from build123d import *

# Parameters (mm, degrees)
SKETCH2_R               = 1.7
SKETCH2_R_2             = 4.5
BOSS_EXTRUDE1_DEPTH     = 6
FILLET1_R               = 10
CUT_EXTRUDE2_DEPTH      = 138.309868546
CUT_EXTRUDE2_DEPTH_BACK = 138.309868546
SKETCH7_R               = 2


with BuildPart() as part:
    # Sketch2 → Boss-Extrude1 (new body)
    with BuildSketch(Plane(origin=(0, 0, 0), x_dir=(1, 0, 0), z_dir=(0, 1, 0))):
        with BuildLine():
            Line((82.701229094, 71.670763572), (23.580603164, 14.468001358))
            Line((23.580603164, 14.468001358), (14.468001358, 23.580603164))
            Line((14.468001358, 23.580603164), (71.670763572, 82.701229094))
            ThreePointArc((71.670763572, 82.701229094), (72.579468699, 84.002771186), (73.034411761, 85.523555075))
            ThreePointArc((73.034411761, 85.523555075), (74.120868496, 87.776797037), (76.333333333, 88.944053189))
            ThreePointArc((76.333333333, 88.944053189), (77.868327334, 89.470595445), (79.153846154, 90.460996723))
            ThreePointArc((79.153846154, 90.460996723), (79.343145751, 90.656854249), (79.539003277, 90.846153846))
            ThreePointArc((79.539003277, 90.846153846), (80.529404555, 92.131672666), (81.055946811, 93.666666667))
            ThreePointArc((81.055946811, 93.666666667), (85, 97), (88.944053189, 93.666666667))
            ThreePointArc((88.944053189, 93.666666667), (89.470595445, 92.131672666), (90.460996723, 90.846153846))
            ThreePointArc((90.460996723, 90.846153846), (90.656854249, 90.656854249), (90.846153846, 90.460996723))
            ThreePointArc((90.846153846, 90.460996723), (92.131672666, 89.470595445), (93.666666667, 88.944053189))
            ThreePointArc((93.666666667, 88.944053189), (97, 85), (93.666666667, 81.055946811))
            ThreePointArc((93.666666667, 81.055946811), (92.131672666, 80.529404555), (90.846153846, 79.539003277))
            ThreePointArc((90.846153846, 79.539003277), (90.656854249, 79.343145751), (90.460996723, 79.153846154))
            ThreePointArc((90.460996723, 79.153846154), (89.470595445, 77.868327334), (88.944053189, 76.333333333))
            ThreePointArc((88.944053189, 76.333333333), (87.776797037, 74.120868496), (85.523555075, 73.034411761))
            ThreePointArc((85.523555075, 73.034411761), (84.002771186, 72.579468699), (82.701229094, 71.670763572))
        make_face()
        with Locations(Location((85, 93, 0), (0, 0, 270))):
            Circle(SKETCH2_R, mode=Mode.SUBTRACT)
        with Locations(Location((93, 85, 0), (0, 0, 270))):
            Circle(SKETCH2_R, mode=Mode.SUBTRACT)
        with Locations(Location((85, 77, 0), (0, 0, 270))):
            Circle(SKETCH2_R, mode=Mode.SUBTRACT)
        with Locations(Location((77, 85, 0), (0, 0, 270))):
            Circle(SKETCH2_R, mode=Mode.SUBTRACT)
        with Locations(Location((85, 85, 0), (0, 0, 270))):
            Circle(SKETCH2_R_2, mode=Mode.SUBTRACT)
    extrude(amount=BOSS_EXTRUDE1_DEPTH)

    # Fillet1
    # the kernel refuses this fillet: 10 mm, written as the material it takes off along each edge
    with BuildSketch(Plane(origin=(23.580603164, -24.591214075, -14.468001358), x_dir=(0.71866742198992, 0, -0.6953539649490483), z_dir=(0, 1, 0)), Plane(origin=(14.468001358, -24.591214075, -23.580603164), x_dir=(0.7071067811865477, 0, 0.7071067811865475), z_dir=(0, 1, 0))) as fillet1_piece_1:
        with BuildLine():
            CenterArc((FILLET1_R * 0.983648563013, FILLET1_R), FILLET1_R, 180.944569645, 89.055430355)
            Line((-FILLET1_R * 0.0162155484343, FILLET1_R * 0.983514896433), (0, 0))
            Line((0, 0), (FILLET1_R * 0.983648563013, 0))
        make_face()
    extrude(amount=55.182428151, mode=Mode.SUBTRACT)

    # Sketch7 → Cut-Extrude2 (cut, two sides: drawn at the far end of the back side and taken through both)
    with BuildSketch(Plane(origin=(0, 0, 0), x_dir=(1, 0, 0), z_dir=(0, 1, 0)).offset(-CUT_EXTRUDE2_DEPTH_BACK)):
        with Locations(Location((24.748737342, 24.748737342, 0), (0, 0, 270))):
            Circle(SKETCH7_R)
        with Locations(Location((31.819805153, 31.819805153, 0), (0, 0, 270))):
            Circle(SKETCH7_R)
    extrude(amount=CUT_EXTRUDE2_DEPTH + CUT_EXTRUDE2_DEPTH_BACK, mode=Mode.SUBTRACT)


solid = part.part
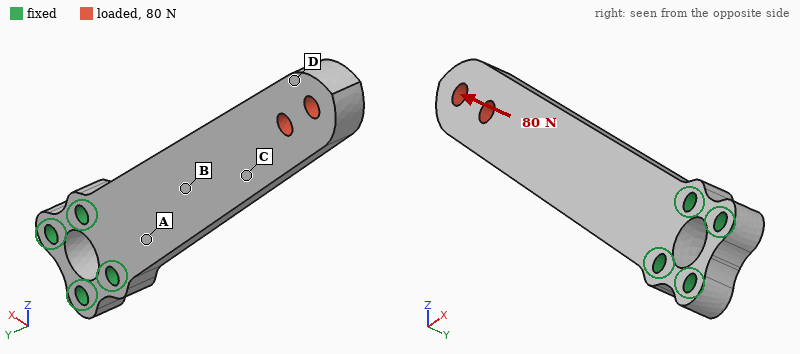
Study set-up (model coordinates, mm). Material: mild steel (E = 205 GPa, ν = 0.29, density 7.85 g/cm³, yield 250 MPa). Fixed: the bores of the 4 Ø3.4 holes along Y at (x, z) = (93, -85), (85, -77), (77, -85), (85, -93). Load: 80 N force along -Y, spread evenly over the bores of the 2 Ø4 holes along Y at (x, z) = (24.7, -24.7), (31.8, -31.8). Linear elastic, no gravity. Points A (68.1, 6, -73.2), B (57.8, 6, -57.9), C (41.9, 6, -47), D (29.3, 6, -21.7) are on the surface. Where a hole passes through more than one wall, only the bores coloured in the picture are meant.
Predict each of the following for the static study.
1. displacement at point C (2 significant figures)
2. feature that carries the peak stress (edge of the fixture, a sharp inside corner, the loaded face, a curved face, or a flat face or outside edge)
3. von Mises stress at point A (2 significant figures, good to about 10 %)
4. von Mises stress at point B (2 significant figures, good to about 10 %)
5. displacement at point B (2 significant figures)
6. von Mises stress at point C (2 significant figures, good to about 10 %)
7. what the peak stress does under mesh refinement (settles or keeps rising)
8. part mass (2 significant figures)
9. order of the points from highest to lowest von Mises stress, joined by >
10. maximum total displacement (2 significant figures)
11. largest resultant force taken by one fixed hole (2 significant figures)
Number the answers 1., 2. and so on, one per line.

1. 0.11 mm
2. edge of the fixture
3. 52 MPa
4. 38 MPa
5. 0.047 mm
6. 22 MPa
7. keeps rising
8. 64 g
9. A > B > C > D
10. 0.24 mm
11. 50 N
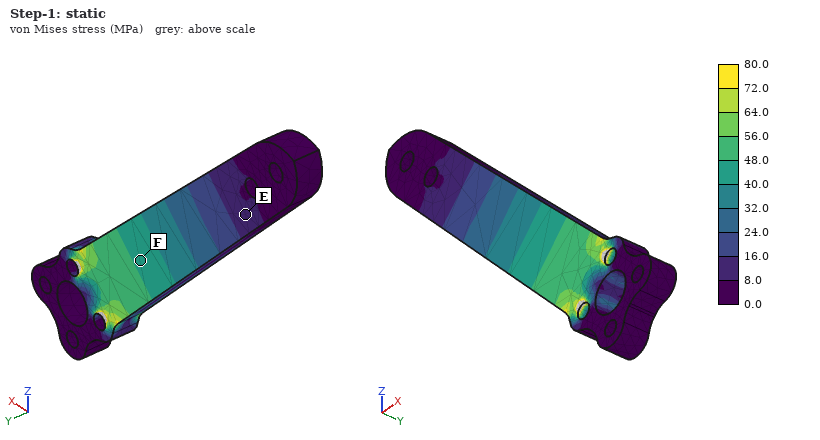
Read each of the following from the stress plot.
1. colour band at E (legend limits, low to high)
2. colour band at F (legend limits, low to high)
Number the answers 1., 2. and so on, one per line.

1. 8.0 to 16.0 MPa
2. 40.0 to 48.0 MPa
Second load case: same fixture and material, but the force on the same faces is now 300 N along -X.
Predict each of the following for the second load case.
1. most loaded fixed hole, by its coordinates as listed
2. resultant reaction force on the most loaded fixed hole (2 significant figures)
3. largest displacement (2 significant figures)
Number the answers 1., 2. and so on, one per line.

1. (85, -77)
2. 1.4 kN
3. 0.10 mm
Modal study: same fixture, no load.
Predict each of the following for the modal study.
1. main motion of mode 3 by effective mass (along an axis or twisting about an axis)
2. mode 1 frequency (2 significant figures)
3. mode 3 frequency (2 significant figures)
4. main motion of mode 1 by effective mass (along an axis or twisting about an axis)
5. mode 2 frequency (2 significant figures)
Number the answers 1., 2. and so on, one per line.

1. along Y
2. 770 Hz
3. 4400 Hz
4. along Y
5. 1900 Hz
